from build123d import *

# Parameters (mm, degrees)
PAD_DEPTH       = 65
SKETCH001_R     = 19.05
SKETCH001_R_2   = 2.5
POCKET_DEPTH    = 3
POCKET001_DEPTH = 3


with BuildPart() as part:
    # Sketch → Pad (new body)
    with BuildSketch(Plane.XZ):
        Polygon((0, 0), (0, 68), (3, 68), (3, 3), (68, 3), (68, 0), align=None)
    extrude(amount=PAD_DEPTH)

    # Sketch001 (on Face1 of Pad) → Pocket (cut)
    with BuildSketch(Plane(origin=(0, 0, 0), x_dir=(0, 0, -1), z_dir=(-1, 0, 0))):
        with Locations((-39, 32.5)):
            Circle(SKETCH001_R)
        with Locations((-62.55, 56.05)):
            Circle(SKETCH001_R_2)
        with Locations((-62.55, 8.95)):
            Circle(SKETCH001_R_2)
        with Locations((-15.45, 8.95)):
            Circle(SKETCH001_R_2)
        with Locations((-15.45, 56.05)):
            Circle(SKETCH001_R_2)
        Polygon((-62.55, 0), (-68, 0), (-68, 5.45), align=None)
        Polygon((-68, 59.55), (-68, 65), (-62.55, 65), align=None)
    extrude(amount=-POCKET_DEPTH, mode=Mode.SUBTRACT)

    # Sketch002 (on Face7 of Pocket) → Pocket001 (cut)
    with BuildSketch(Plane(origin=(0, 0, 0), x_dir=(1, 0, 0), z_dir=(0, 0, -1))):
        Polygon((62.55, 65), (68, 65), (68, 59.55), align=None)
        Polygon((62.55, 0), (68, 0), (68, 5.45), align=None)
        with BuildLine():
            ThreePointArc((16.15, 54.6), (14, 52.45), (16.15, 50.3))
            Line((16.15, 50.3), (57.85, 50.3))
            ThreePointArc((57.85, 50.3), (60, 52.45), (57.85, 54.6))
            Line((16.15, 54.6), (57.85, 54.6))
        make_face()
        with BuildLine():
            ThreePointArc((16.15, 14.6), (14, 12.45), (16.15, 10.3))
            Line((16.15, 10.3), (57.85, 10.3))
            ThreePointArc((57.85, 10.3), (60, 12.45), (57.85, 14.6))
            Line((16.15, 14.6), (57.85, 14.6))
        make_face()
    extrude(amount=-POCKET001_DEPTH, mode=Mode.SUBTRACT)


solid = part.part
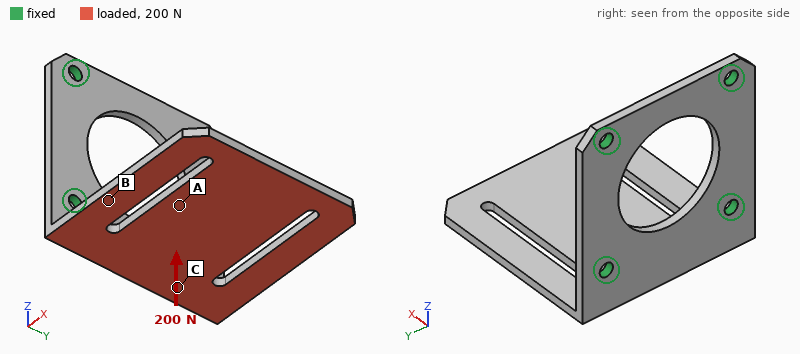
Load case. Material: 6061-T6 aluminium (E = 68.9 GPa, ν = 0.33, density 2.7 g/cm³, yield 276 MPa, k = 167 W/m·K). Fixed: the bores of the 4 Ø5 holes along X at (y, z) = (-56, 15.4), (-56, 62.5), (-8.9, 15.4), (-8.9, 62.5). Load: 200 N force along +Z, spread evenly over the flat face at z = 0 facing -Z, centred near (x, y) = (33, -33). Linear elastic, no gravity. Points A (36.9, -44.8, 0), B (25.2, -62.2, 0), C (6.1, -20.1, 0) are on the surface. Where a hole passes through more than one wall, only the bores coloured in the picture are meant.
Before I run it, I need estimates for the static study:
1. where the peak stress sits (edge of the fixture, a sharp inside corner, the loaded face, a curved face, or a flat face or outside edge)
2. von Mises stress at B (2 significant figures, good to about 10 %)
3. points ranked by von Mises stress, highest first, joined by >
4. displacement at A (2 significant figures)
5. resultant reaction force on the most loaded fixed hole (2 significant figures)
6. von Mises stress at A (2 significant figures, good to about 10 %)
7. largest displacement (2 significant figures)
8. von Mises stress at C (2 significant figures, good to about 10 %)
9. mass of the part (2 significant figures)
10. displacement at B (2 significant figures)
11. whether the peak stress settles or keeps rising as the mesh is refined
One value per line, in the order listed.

edge of the fixture
33 MPa
C > B > A
0.58 mm
110 N
16 MPa
1.3 mm
53 MPa
57 g
0.34 mm
keeps rising
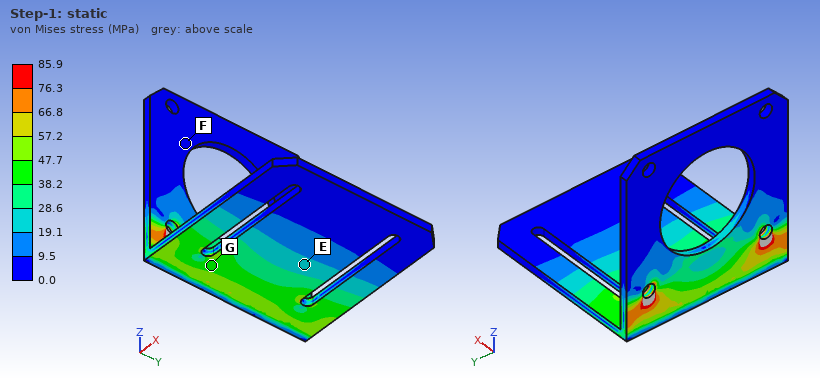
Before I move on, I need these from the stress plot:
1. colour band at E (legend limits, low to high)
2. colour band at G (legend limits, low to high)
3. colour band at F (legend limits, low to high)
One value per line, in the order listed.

19.1 to 28.6 MPa
38.2 to 47.7 MPa
0.0 to 9.5 MPa
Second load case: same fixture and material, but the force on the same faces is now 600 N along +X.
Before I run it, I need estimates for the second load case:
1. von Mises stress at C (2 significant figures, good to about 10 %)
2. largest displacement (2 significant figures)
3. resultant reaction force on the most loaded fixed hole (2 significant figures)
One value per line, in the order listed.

12 MPa
0.62 mm
310 N
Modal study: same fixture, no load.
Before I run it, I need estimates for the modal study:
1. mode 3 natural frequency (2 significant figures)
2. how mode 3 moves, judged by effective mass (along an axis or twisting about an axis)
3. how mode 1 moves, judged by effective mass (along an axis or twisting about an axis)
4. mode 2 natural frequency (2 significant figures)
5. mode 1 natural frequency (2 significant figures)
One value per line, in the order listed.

2000 Hz
along Y
along Z
1200 Hz
430 Hz
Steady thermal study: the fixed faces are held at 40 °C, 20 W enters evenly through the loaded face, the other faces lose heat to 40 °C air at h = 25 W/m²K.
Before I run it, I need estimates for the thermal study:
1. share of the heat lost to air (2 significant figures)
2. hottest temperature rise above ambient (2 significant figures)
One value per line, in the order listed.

16 %
28 K
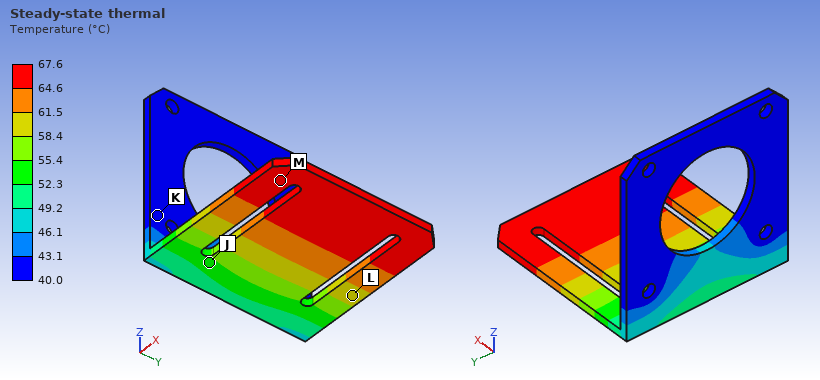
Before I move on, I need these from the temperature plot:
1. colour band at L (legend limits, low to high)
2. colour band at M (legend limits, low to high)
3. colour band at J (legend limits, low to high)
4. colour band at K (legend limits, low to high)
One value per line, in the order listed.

58.4 to 61.5 °C
64.6 to 67.6 °C
52.3 to 55.4 °C
40.0 to 43.1 °C
